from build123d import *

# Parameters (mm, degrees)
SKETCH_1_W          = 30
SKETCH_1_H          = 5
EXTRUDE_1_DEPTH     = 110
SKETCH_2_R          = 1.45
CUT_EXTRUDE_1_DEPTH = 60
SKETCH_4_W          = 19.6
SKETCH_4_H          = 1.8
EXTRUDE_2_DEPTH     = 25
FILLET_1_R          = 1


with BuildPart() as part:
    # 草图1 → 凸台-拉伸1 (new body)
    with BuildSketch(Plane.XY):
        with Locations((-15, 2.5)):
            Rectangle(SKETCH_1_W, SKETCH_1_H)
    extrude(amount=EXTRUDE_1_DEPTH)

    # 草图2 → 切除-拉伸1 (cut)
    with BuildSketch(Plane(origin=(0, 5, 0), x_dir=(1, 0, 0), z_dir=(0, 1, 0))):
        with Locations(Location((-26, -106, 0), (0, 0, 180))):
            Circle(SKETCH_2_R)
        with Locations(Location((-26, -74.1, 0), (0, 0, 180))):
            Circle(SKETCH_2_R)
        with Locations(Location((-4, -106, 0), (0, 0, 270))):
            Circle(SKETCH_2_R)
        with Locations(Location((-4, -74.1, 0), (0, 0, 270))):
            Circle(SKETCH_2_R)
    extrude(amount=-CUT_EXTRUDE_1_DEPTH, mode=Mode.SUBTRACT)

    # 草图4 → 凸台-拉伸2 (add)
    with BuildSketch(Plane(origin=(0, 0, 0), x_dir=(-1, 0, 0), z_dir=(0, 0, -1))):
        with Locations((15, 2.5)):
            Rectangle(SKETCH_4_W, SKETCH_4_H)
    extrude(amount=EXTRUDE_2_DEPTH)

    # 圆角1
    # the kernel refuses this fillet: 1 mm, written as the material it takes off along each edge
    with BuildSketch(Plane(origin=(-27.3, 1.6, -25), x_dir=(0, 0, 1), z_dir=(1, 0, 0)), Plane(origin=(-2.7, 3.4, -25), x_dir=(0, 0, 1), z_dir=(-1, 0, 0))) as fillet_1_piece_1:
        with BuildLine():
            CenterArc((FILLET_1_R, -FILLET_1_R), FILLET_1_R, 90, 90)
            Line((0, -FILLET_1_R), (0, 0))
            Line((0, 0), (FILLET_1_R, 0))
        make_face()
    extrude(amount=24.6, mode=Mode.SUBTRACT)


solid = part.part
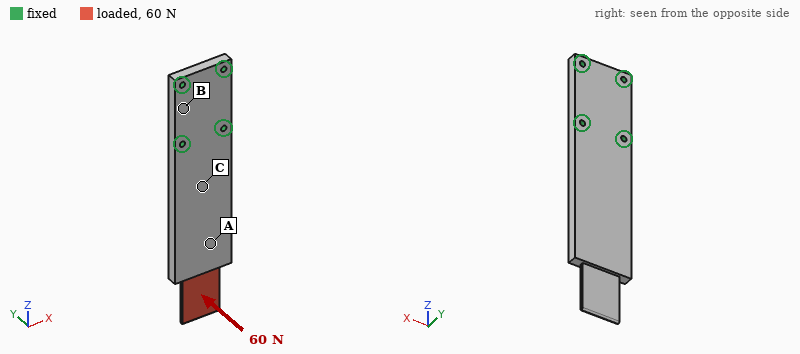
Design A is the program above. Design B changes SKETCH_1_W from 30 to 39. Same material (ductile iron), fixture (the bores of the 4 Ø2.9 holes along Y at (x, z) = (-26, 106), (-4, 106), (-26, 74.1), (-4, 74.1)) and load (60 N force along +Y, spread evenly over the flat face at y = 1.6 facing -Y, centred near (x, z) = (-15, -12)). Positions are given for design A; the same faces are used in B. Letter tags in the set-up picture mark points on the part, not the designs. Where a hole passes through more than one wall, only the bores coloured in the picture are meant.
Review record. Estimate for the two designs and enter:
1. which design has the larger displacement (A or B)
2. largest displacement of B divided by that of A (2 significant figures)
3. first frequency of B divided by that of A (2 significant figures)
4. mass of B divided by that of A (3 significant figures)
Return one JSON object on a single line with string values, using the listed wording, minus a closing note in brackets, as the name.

{"which design has the larger displacement": "A", "largest displacement of B divided by that of A": "0.82", "first frequency of B divided by that of A": "1.0", "mass of B divided by that of A": "1.29"}
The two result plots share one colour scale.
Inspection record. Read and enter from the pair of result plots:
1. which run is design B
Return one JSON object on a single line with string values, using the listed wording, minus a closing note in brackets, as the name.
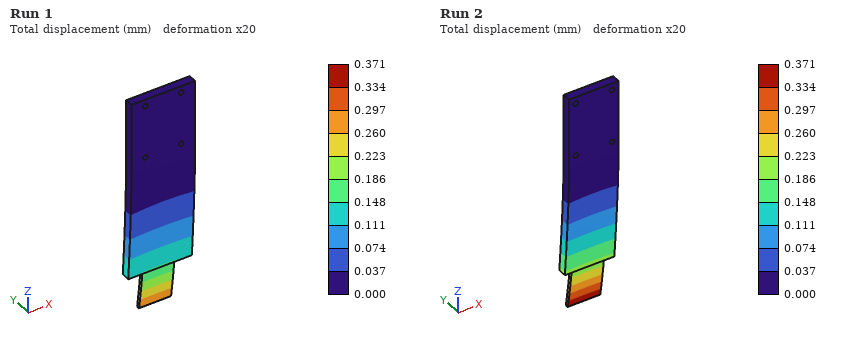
{"which run is design B": "Run 1"}
